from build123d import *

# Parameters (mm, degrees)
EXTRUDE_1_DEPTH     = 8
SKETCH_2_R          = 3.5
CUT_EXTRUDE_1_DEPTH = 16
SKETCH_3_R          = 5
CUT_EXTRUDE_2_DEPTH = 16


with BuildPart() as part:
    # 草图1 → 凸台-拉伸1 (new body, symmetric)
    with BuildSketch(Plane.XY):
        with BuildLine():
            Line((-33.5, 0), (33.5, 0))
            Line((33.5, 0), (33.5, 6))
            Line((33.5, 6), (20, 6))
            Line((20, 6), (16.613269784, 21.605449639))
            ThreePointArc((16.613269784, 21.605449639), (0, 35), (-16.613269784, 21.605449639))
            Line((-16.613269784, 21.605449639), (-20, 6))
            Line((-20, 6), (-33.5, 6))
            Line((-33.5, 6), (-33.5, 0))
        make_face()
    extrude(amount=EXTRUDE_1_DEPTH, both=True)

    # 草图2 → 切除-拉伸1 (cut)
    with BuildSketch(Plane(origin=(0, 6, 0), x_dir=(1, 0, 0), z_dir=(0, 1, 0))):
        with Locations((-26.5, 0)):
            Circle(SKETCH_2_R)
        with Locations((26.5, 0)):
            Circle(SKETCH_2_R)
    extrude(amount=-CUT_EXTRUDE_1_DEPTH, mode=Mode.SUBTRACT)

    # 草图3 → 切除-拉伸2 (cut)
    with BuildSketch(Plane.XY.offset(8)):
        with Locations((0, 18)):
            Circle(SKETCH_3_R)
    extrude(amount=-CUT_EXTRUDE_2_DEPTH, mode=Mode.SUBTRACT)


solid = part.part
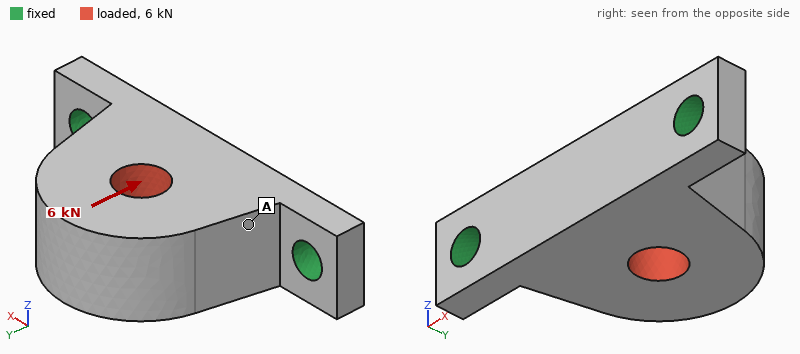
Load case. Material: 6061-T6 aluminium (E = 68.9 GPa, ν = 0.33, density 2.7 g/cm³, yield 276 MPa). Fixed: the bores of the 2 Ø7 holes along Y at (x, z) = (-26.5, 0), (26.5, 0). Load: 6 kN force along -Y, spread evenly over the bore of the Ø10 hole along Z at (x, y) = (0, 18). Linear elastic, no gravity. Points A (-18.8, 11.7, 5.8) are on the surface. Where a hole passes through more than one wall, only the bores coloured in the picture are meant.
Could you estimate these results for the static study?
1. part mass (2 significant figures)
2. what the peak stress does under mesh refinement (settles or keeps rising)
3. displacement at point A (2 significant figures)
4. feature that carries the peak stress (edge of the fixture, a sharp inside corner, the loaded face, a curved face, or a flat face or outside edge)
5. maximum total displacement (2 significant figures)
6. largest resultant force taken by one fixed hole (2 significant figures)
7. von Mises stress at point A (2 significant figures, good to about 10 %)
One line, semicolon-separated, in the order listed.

52 g; keeps rising; 17 µm; edge of the fixture; 25 µm; 3.5 kN; 34 MPa
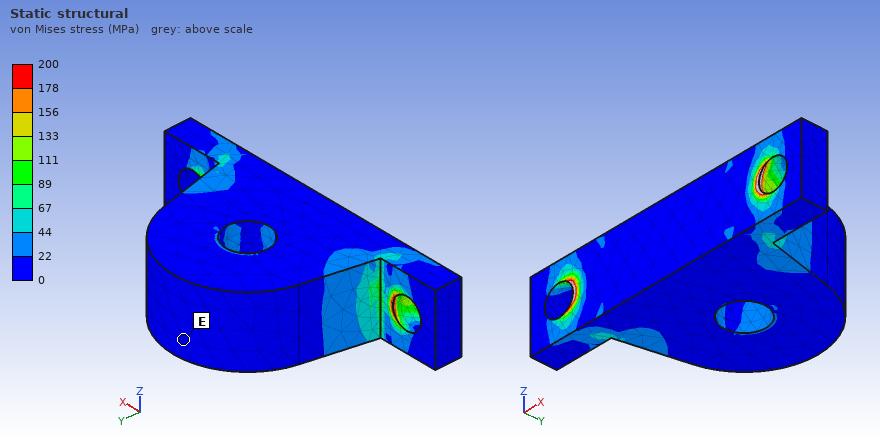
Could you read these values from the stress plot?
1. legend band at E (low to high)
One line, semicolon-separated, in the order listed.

0 to 22 MPa
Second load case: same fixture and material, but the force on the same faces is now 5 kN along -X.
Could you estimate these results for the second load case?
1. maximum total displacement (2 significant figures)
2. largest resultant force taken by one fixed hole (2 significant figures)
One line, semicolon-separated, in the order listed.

21 µm; 3.0 kN
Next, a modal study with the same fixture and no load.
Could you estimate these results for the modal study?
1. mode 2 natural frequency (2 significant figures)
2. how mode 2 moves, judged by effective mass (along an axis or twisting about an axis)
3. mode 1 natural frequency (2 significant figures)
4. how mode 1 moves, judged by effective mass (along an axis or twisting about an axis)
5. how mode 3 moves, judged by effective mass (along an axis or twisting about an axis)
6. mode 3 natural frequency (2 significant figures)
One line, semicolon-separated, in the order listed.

13 kHz; along Y; 4100 Hz; along Z; along X; 14 kHz
